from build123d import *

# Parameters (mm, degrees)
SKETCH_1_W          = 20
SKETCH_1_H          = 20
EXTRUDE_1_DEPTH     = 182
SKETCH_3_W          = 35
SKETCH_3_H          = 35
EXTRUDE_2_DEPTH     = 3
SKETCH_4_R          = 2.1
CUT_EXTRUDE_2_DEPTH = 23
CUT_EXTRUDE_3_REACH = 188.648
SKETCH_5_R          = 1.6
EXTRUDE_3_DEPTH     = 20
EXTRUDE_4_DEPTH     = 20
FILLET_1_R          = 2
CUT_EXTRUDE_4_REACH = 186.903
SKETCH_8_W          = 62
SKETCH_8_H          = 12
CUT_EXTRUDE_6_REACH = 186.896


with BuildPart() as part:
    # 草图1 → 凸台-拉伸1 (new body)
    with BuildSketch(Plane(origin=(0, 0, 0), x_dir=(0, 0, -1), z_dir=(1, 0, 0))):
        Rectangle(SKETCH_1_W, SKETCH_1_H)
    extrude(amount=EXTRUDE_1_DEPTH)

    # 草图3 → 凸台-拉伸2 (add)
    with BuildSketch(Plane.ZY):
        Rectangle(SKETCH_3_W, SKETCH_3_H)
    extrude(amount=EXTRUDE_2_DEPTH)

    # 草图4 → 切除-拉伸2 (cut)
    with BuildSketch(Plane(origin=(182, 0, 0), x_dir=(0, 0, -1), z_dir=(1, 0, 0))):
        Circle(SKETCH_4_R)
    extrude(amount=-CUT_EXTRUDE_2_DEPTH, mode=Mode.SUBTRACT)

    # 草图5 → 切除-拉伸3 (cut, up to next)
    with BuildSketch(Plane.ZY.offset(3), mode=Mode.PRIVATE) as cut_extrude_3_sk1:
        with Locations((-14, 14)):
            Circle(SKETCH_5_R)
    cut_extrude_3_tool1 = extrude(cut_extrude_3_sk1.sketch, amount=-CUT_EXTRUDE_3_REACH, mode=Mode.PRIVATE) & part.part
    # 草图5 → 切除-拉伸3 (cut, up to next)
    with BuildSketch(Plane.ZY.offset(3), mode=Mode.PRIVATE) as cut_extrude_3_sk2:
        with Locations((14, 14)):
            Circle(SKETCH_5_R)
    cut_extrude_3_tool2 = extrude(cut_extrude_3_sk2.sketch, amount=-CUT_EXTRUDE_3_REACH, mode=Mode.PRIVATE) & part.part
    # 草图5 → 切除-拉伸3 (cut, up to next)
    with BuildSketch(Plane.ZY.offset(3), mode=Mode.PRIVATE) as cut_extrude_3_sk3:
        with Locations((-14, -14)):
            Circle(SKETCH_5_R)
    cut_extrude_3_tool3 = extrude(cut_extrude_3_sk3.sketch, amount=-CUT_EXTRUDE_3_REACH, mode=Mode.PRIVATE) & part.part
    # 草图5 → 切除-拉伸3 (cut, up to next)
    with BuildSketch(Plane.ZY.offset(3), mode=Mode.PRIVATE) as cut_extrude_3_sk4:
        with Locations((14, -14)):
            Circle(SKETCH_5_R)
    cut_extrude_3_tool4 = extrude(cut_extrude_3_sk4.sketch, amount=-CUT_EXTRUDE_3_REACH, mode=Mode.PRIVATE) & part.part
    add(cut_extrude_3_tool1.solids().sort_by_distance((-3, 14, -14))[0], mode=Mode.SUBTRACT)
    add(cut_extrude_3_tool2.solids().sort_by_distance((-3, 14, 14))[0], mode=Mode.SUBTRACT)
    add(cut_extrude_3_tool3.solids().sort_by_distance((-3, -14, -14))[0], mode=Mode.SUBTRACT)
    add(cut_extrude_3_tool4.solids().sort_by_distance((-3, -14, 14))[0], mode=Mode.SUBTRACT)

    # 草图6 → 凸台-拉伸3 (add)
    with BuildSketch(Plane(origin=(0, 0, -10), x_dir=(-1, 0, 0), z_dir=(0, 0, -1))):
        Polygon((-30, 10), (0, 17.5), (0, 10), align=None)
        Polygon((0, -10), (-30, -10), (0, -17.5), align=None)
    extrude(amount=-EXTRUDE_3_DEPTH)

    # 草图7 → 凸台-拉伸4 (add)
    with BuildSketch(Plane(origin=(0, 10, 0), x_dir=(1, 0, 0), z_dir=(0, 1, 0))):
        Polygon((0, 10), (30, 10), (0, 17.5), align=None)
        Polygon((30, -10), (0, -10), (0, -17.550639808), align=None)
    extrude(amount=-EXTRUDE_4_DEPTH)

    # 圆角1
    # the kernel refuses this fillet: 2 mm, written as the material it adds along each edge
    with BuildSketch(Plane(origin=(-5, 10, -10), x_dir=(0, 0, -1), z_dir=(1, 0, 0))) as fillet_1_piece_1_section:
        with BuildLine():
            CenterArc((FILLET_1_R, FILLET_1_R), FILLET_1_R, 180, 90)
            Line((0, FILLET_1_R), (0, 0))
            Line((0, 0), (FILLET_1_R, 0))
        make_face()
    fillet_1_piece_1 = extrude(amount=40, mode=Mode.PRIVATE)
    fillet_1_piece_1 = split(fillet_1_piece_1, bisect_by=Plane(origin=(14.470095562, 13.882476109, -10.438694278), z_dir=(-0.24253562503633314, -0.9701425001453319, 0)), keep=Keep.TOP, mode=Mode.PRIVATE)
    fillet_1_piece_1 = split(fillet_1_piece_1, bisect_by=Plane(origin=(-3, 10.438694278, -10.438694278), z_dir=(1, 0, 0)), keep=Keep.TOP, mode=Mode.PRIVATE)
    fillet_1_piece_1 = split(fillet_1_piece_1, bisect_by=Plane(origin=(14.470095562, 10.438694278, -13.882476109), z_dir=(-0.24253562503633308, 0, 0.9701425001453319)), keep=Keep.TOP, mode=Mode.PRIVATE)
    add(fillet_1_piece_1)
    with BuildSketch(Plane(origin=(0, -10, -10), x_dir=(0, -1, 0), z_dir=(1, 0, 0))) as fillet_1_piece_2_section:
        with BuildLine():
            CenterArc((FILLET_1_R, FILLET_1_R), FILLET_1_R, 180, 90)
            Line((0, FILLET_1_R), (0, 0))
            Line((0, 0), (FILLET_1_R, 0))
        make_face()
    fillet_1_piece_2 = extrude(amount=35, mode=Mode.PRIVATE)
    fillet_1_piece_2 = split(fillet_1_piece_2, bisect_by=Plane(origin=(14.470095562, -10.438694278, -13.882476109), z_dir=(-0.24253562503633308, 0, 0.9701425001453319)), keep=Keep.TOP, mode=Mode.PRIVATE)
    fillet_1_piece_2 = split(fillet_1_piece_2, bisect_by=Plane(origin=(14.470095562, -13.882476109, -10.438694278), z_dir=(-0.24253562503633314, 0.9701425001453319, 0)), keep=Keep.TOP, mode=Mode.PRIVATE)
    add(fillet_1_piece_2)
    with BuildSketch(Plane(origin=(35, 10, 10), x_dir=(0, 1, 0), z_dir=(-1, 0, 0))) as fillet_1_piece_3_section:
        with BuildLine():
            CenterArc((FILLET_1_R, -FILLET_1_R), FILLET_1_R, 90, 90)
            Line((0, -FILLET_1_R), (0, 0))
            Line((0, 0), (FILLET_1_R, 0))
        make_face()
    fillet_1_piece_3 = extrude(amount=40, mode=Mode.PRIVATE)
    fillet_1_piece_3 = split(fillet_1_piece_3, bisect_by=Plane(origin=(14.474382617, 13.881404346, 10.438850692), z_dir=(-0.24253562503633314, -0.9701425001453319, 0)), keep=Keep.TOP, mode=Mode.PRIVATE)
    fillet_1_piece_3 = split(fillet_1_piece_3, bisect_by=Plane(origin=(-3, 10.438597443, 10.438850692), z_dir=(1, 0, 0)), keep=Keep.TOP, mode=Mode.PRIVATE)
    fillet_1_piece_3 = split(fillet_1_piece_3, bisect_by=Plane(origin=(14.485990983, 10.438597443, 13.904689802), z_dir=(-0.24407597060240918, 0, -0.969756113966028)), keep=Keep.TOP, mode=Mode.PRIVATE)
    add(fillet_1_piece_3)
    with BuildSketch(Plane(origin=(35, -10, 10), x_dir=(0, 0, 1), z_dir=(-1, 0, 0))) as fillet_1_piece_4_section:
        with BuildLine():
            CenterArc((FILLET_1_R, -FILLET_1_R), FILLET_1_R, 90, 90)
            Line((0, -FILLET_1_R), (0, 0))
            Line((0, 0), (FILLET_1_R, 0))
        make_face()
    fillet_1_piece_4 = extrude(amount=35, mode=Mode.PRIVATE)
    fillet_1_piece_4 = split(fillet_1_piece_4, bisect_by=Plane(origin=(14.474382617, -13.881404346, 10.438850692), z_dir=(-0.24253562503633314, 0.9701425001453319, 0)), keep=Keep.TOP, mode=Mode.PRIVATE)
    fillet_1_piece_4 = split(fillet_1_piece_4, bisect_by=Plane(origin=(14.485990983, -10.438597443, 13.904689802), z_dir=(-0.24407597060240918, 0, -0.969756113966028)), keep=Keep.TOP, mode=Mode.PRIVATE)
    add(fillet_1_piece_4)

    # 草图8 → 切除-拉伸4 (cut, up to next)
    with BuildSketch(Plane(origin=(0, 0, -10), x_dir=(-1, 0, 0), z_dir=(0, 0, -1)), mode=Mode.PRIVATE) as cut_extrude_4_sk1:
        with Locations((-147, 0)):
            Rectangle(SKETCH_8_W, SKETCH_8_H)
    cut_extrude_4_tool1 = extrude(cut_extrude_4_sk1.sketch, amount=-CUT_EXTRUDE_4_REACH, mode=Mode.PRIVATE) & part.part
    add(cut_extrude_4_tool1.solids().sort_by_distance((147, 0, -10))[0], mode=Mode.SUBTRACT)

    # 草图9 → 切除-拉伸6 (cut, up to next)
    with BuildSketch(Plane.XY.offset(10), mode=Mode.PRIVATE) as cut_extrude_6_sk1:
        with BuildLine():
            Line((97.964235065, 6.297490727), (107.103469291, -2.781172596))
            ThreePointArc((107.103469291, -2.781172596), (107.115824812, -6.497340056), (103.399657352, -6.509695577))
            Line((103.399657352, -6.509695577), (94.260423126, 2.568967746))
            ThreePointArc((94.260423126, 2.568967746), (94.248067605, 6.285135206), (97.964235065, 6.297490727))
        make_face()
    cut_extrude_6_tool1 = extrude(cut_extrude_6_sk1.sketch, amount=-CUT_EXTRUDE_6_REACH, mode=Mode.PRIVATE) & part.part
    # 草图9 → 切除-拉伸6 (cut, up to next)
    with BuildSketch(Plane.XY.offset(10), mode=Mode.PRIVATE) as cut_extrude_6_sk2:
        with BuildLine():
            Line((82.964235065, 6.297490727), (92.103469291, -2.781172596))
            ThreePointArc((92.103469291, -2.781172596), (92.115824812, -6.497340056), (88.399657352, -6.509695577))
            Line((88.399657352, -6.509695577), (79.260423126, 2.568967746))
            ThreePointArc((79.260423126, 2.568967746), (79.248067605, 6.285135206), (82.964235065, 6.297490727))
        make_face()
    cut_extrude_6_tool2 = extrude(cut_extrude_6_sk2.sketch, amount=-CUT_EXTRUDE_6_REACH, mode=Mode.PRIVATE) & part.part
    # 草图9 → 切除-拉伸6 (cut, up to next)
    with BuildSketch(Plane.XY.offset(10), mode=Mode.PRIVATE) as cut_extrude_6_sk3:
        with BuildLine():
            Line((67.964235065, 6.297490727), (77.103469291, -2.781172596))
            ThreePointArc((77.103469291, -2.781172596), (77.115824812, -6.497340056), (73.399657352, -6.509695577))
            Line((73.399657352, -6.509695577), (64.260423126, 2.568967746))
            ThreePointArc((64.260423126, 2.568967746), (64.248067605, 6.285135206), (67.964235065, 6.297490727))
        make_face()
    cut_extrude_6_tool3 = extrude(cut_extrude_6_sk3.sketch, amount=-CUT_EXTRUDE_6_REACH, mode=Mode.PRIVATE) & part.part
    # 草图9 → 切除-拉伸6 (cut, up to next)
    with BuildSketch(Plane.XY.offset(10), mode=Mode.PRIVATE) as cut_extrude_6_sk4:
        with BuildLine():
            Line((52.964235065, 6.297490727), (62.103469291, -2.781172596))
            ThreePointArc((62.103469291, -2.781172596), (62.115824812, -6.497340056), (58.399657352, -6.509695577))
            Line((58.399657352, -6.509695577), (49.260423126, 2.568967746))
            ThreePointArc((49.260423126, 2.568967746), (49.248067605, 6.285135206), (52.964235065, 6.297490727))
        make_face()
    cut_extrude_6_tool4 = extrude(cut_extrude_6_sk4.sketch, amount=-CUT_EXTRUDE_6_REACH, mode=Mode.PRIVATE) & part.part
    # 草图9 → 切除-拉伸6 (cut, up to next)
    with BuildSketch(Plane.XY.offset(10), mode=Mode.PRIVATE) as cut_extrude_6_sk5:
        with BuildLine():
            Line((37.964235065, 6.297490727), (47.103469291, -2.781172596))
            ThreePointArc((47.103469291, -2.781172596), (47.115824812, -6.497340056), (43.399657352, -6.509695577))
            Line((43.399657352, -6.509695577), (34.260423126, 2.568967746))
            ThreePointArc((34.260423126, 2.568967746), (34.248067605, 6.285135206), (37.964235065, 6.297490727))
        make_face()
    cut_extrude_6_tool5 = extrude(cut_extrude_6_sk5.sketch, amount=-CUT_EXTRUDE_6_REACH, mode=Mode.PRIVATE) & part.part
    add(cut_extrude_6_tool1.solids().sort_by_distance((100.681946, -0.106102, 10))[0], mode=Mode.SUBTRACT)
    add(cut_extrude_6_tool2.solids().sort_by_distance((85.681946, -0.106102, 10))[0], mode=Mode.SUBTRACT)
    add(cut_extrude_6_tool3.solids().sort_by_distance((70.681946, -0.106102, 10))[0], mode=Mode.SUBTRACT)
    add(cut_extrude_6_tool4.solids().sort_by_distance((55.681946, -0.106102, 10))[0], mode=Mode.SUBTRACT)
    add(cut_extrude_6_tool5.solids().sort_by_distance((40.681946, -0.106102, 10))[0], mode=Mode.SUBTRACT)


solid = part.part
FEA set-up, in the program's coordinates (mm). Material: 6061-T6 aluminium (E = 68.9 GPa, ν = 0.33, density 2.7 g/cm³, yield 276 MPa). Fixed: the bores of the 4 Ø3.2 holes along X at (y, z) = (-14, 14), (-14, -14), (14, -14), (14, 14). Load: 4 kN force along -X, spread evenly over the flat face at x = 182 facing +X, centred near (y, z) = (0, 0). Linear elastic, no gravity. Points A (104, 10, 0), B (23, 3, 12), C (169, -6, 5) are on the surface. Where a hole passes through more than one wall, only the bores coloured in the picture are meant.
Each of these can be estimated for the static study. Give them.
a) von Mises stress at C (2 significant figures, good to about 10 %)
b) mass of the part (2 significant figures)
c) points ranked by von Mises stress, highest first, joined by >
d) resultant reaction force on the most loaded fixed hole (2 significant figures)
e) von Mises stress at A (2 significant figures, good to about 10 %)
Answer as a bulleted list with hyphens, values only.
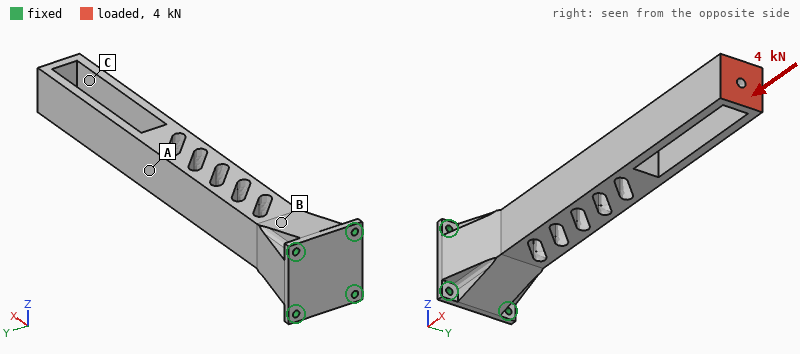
- 45 MPa
- 170 g
- C > A > B
- 1.1 kN
- 29 MPa
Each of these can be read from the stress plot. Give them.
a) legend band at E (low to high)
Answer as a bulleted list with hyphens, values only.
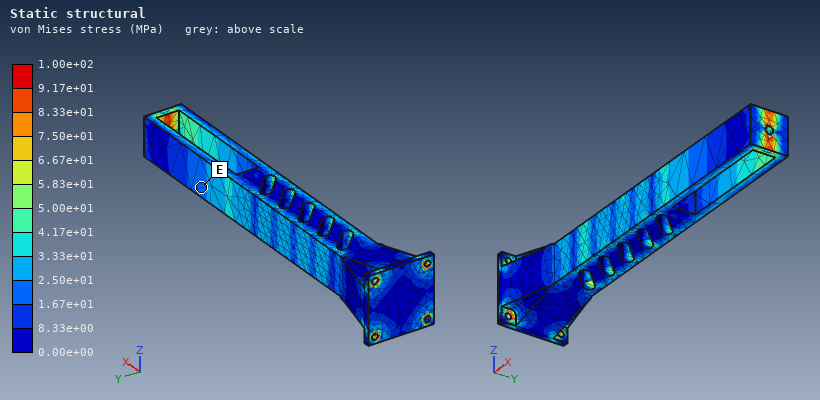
- 1.67e+01 to 2.50e+01 MPa
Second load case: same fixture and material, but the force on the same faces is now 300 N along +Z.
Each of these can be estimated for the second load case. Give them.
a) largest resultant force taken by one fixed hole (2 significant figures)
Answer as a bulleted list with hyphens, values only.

- 1.1 kN
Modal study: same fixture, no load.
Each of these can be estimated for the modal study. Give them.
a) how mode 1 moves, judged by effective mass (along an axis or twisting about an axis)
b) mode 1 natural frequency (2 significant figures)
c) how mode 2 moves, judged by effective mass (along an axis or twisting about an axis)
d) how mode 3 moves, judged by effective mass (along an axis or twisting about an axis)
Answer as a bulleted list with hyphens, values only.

- along Z
- 530 Hz
- along Y
- along Y
